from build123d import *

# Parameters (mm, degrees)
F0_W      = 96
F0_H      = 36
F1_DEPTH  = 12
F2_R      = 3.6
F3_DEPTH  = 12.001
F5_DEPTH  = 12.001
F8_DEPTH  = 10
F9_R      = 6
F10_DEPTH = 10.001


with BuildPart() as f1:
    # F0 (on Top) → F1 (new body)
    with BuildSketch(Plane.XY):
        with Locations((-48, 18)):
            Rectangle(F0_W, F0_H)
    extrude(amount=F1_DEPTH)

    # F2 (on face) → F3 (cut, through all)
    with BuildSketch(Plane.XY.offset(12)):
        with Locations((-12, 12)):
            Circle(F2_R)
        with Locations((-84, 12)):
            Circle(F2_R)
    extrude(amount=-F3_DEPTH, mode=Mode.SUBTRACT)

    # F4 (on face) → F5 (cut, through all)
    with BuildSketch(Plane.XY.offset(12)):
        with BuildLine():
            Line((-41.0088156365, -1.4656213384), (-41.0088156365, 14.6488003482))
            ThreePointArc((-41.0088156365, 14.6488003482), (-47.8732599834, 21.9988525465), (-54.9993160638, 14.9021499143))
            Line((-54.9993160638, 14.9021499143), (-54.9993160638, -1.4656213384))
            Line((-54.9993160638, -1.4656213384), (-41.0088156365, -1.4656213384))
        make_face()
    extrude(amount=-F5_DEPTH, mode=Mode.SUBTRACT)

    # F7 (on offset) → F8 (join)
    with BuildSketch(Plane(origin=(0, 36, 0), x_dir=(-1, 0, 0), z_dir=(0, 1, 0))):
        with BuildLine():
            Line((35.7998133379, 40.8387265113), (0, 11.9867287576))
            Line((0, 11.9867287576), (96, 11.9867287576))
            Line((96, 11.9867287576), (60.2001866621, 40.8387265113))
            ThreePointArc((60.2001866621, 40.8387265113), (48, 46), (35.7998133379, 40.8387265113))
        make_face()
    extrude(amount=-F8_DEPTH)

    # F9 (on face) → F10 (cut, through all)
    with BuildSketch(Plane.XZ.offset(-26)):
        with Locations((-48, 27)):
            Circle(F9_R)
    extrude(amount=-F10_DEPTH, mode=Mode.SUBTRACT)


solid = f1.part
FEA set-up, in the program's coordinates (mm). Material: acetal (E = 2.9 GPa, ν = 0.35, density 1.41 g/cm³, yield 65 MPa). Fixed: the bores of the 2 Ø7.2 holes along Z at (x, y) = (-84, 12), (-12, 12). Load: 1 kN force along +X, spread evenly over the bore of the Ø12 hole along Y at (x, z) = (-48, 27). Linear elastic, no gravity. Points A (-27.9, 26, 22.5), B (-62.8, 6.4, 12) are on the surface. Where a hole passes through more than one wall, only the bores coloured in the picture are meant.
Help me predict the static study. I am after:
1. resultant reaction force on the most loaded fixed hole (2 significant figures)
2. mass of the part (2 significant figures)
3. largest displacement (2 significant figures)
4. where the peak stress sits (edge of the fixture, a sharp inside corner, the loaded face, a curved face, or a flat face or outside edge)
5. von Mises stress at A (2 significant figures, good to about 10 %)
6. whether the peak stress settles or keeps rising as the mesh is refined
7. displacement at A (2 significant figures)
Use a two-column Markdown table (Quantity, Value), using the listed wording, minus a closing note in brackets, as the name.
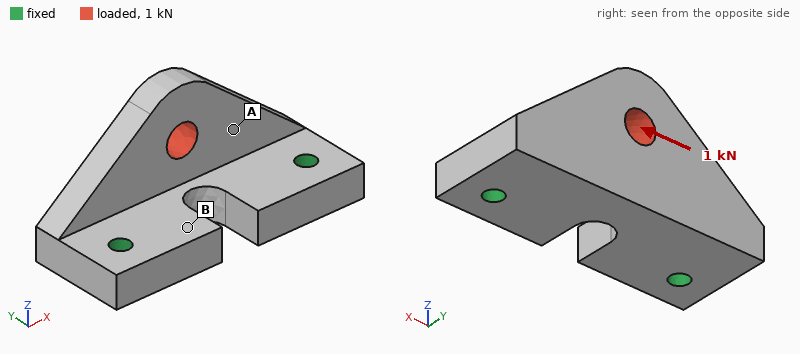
| Quantity | Value |
|---|---|
| resultant reaction force on the most loaded fixed hole | 610 N |
| mass of the part | 76 g |
| largest displacement | 0.12 mm |
| where the peak stress sits | edge of the fixture |
| von Mises stress at A | 3.5 MPa |
| whether the peak stress settles or keeps rising as the mesh is refined | keeps rising |
| displacement at A | 0.075 mm |
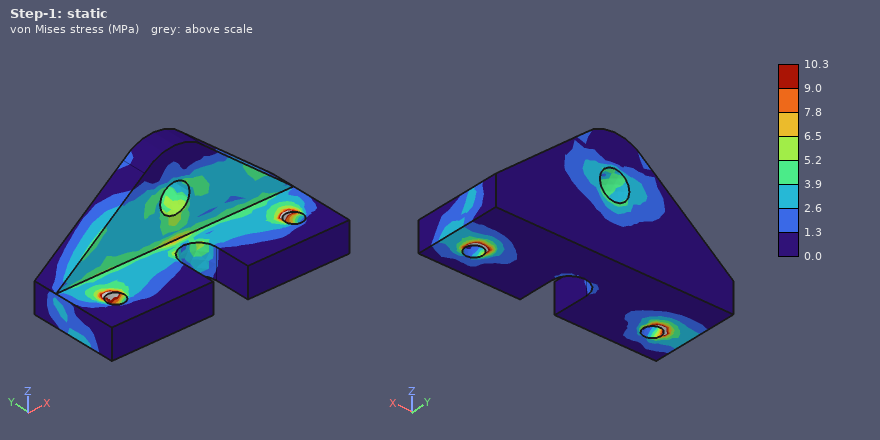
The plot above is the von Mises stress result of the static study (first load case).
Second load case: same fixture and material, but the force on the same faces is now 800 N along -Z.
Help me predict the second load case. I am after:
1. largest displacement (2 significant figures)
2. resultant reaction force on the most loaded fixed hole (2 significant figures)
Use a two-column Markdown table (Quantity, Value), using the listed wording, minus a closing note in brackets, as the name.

| Quantity | Value |
|---|---|
| largest displacement | 0.33 mm |
| resultant reaction force on the most loaded fixed hole | 400 N |
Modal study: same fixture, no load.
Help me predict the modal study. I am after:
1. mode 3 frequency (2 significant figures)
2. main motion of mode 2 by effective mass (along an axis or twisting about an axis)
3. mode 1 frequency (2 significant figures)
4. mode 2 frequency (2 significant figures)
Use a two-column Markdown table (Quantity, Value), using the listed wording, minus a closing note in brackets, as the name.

| Quantity | Value |
|---|---|
| mode 3 frequency | 2700 Hz |
| main motion of mode 2 by effective mass | along Z |
| mode 1 frequency | 1300 Hz |
| mode 2 frequency | 2600 Hz |
